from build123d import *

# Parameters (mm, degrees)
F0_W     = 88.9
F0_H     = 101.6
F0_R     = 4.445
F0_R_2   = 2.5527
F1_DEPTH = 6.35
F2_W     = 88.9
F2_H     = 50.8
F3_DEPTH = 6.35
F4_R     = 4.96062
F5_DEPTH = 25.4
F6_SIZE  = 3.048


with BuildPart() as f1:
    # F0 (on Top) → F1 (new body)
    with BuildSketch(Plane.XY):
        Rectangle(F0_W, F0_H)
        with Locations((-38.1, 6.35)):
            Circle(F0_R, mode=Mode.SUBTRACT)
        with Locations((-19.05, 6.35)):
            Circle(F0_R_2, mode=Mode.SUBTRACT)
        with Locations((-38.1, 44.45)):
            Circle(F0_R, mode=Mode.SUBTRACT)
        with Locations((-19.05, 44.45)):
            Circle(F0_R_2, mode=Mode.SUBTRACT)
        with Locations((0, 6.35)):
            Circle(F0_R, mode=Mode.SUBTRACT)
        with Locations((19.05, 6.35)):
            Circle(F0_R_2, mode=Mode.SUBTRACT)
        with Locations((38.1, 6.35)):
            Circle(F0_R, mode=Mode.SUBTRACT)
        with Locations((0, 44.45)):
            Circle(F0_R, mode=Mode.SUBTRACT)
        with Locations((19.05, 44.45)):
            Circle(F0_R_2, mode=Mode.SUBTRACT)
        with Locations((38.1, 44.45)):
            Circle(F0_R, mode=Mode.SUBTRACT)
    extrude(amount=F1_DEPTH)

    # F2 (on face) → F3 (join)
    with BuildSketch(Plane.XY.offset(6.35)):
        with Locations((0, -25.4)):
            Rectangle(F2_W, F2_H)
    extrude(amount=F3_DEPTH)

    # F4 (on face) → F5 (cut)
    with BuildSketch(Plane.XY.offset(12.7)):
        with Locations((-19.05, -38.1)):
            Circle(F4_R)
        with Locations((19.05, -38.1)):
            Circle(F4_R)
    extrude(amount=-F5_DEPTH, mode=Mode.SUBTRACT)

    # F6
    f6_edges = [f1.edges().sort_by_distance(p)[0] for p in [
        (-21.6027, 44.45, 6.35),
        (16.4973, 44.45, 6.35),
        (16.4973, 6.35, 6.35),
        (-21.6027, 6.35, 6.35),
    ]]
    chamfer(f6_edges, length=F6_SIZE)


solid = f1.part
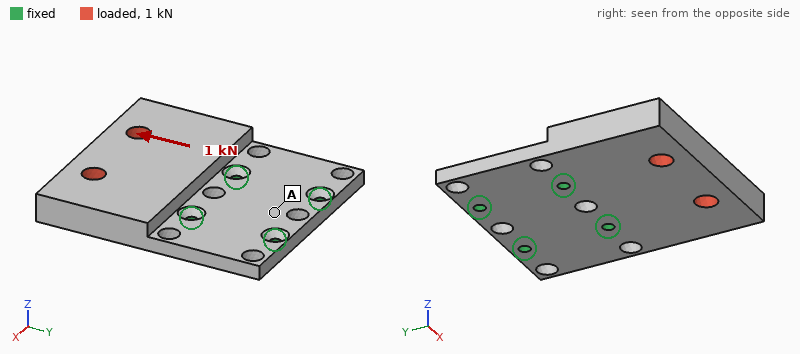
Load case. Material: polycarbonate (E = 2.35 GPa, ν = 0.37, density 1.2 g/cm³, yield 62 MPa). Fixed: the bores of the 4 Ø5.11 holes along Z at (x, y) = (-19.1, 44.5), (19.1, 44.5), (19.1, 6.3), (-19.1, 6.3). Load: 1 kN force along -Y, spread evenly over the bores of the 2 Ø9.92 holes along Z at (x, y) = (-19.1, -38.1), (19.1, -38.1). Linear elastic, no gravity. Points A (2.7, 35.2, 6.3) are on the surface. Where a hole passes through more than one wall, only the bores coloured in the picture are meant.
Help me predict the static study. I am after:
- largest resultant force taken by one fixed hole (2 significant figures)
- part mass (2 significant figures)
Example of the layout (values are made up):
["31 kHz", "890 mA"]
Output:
["330 N", "97 g"]
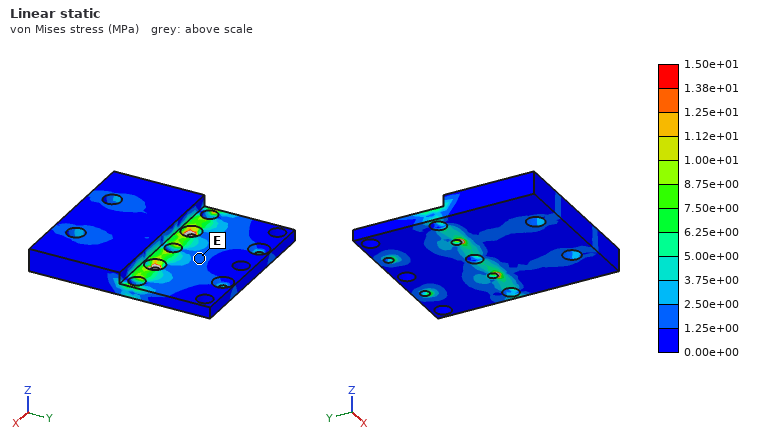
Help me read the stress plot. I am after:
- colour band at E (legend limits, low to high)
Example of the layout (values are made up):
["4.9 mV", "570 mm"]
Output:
["1.25e+00 to 2.50e+00 MPa"]
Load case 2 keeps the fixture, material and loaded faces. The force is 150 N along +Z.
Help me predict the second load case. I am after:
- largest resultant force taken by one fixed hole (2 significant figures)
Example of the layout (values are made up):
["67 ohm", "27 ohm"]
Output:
["170 N"]
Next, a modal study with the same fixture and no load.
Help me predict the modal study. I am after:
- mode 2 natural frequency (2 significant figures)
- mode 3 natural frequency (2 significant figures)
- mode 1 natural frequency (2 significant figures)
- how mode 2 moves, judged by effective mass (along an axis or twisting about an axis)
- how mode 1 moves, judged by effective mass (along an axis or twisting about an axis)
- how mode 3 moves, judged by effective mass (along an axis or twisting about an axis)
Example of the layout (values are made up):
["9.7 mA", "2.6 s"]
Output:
["790 Hz", "1600 Hz", "290 Hz", "twisting about Y", "along Z", "along X"]
